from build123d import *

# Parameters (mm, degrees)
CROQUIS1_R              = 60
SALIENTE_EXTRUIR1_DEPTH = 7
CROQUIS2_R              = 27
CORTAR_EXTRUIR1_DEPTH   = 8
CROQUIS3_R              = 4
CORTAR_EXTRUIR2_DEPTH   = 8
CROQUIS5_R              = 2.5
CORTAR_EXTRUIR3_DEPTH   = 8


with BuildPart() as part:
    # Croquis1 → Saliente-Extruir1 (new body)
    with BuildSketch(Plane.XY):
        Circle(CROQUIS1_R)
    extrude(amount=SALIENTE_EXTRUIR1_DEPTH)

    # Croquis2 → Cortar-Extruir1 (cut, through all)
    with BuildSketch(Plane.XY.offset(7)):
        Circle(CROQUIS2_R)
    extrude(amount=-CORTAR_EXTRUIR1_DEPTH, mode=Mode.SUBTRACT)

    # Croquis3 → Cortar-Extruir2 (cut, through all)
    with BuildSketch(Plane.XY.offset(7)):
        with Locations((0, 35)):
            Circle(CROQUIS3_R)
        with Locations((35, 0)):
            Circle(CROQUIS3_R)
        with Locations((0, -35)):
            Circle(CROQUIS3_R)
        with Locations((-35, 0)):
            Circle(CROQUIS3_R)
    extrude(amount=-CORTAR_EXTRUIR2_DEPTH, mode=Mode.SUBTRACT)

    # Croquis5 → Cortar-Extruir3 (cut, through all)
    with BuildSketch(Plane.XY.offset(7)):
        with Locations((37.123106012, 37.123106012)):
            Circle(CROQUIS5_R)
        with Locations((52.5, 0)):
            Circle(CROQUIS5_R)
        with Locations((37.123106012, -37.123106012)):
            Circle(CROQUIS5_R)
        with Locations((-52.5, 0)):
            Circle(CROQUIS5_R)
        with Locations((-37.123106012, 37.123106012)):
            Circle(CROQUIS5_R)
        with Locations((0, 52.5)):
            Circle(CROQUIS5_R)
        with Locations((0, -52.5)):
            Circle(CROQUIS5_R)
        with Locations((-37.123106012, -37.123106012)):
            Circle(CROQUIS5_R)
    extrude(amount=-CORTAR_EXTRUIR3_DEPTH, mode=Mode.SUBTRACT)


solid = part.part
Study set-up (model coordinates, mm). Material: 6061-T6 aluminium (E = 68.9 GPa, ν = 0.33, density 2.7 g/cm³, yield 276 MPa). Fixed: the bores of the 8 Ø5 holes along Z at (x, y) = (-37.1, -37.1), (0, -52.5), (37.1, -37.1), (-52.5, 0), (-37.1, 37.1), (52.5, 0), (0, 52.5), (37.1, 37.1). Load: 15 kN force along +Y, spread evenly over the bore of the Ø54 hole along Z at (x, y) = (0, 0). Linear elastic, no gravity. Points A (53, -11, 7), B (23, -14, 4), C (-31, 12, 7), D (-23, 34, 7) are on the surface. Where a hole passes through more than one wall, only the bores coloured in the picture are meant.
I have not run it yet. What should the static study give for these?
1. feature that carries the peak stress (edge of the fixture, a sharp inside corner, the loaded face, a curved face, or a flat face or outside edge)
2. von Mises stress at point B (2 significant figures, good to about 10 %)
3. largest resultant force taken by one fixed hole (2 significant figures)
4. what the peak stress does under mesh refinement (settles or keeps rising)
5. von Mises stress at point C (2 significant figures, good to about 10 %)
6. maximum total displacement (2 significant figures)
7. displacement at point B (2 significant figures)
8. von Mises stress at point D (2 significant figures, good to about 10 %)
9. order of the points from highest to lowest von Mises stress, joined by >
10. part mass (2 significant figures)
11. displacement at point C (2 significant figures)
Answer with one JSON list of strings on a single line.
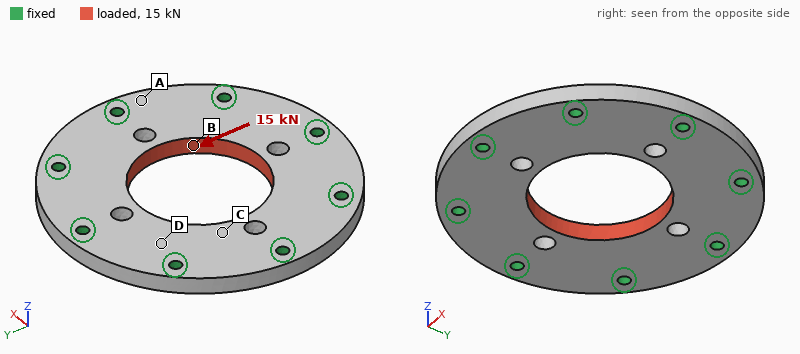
["edge of the fixture", "20 MPa", "2.7 kN", "keeps rising", "16 MPa", "10 µm", "7.5 µm", "8.3 MPa", "B > C > D > A", "160 g", "5.2 µm"]
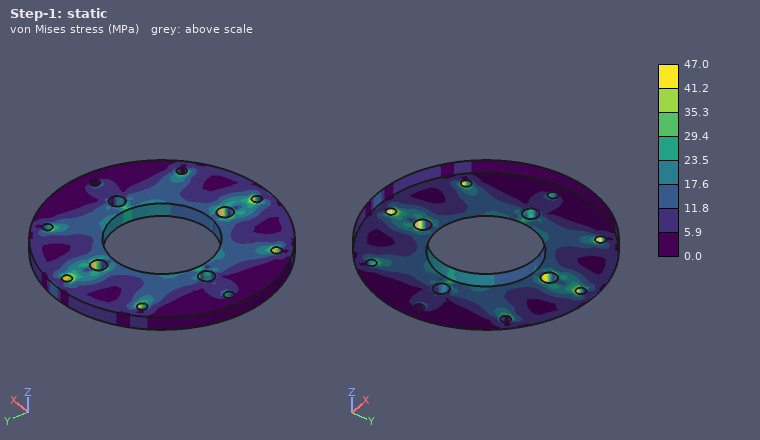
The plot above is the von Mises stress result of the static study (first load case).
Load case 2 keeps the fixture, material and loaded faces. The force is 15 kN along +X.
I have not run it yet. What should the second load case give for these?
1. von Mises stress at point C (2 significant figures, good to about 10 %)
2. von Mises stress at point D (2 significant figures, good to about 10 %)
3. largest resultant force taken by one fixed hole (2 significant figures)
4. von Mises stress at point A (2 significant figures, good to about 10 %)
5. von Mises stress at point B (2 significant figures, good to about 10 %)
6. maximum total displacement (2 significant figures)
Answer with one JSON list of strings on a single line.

["12 MPa", "14 MPa", "2.7 kN", "7.5 MPa", "15 MPa", "10 µm"]
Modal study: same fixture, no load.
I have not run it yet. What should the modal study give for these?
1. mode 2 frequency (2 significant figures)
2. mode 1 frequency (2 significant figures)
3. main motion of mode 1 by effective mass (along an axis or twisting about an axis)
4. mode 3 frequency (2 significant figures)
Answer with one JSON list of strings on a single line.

["10 kHz", "8500 Hz", "along Z", "10 kHz"]
